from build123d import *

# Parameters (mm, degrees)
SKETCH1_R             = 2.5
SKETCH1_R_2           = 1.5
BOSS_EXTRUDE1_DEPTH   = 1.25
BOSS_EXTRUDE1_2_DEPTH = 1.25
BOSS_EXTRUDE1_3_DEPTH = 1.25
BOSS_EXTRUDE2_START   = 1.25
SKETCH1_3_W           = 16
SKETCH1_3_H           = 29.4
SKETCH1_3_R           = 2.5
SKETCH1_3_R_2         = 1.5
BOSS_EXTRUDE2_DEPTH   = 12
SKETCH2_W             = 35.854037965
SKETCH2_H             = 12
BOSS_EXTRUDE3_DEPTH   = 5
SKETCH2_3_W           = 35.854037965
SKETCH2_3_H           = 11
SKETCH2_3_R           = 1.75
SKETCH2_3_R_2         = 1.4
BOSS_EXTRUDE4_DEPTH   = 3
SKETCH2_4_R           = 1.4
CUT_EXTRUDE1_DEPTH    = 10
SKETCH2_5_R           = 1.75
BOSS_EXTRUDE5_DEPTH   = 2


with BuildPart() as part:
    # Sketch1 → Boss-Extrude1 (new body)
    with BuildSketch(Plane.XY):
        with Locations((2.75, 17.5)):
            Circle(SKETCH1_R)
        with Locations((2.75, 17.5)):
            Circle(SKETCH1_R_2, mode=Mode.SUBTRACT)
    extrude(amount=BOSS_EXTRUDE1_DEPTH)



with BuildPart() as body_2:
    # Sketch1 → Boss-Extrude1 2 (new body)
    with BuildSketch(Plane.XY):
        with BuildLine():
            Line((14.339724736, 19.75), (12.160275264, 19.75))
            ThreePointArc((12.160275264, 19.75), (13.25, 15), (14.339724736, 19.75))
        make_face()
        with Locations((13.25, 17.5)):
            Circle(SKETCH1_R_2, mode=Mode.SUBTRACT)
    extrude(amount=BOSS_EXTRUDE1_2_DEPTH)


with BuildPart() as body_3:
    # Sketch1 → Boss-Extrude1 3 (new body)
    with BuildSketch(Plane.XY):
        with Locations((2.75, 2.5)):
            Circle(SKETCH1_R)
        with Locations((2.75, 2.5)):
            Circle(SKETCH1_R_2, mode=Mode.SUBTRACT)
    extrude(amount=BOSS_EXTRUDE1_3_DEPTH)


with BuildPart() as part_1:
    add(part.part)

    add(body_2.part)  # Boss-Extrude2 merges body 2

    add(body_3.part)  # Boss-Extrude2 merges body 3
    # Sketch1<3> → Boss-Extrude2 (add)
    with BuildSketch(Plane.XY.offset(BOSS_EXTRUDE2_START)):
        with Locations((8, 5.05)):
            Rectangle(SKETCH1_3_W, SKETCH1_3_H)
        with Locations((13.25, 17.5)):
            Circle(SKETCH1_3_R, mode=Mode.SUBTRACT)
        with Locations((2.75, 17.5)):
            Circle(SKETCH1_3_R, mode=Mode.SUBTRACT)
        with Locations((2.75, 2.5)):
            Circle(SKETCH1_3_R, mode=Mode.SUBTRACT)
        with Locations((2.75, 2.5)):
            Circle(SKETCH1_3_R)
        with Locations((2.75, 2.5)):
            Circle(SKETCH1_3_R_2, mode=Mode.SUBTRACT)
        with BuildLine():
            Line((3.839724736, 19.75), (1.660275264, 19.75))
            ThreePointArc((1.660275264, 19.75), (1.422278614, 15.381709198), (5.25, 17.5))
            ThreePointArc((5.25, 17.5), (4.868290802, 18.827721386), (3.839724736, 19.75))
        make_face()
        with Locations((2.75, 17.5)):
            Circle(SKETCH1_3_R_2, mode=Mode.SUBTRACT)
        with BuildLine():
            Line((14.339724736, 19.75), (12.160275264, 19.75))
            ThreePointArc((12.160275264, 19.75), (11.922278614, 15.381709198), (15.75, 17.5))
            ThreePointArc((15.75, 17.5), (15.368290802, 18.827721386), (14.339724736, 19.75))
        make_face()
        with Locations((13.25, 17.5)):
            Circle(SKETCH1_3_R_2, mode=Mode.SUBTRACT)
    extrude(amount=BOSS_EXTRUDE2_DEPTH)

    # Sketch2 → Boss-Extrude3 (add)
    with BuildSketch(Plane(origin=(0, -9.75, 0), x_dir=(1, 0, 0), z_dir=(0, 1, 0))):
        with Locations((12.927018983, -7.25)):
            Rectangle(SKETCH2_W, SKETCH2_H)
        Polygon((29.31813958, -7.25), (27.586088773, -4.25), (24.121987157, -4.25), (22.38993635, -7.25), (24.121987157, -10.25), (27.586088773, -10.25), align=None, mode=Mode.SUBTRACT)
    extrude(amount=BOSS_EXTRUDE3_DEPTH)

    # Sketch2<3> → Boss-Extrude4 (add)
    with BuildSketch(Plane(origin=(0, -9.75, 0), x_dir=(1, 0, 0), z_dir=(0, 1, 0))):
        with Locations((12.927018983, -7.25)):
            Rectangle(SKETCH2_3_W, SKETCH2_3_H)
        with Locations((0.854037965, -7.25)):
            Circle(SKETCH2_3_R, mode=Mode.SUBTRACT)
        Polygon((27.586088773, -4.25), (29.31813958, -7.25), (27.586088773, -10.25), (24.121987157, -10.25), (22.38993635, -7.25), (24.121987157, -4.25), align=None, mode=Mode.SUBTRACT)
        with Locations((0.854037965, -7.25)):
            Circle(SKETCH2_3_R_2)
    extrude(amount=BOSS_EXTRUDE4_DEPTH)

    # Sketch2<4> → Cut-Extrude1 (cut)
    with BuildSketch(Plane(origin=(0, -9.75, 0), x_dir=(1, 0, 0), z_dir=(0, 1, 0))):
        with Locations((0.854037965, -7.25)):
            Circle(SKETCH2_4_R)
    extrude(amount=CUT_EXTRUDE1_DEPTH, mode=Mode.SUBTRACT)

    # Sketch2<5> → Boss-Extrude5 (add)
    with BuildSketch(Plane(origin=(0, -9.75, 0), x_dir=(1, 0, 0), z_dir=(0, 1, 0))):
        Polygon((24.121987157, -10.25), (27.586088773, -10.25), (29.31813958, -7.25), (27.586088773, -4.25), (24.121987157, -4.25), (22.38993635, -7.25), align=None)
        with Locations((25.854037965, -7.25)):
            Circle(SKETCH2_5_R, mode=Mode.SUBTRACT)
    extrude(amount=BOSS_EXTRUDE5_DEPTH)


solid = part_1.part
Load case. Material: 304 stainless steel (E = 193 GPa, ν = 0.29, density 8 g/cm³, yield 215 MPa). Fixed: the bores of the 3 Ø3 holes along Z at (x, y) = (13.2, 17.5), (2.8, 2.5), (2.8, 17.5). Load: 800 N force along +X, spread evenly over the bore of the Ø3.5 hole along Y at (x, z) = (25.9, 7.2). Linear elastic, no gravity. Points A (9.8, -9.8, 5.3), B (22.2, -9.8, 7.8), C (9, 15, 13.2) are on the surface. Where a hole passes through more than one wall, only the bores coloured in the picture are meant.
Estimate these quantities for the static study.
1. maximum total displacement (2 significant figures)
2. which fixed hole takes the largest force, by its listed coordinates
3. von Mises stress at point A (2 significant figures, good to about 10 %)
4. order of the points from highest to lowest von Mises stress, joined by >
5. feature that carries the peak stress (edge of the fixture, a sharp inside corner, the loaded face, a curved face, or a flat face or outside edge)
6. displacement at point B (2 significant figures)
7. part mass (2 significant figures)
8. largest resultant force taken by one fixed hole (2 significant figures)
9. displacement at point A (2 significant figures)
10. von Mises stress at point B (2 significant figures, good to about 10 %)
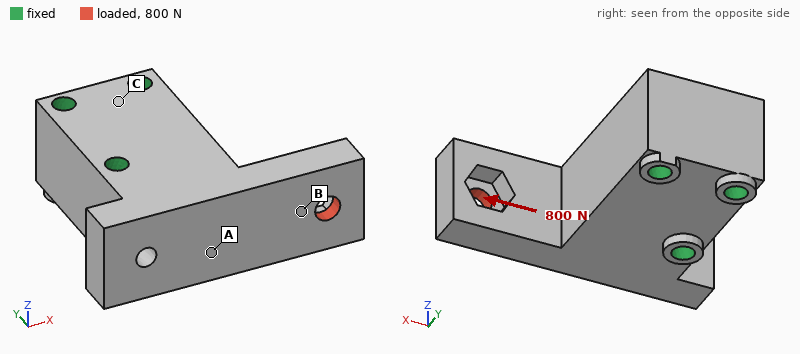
12 µm
(2.8, 2.5)
15 MPa
B > A > C
the loaded face
6.1 µm
52 g
1.1 kN
2.0 µm
45 MPa
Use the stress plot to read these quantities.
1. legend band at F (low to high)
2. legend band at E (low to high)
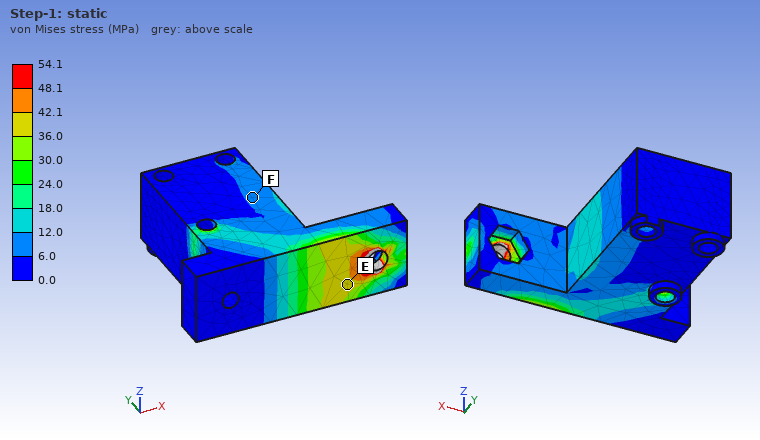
6.0 to 12.0 MPa
36.0 to 42.1 MPa
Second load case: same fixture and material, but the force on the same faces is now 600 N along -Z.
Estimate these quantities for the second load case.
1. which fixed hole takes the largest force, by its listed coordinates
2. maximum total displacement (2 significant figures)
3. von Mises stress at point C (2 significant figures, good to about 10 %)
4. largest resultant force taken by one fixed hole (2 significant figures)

(2.8, 2.5)
22 µm
9.1 MPa
480 N
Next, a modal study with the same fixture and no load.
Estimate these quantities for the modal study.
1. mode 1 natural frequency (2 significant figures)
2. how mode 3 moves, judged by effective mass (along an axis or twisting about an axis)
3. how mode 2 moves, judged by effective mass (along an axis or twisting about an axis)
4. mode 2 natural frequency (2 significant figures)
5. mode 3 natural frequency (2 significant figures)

12 kHz
along X
along Z
13 kHz
26 kHz
